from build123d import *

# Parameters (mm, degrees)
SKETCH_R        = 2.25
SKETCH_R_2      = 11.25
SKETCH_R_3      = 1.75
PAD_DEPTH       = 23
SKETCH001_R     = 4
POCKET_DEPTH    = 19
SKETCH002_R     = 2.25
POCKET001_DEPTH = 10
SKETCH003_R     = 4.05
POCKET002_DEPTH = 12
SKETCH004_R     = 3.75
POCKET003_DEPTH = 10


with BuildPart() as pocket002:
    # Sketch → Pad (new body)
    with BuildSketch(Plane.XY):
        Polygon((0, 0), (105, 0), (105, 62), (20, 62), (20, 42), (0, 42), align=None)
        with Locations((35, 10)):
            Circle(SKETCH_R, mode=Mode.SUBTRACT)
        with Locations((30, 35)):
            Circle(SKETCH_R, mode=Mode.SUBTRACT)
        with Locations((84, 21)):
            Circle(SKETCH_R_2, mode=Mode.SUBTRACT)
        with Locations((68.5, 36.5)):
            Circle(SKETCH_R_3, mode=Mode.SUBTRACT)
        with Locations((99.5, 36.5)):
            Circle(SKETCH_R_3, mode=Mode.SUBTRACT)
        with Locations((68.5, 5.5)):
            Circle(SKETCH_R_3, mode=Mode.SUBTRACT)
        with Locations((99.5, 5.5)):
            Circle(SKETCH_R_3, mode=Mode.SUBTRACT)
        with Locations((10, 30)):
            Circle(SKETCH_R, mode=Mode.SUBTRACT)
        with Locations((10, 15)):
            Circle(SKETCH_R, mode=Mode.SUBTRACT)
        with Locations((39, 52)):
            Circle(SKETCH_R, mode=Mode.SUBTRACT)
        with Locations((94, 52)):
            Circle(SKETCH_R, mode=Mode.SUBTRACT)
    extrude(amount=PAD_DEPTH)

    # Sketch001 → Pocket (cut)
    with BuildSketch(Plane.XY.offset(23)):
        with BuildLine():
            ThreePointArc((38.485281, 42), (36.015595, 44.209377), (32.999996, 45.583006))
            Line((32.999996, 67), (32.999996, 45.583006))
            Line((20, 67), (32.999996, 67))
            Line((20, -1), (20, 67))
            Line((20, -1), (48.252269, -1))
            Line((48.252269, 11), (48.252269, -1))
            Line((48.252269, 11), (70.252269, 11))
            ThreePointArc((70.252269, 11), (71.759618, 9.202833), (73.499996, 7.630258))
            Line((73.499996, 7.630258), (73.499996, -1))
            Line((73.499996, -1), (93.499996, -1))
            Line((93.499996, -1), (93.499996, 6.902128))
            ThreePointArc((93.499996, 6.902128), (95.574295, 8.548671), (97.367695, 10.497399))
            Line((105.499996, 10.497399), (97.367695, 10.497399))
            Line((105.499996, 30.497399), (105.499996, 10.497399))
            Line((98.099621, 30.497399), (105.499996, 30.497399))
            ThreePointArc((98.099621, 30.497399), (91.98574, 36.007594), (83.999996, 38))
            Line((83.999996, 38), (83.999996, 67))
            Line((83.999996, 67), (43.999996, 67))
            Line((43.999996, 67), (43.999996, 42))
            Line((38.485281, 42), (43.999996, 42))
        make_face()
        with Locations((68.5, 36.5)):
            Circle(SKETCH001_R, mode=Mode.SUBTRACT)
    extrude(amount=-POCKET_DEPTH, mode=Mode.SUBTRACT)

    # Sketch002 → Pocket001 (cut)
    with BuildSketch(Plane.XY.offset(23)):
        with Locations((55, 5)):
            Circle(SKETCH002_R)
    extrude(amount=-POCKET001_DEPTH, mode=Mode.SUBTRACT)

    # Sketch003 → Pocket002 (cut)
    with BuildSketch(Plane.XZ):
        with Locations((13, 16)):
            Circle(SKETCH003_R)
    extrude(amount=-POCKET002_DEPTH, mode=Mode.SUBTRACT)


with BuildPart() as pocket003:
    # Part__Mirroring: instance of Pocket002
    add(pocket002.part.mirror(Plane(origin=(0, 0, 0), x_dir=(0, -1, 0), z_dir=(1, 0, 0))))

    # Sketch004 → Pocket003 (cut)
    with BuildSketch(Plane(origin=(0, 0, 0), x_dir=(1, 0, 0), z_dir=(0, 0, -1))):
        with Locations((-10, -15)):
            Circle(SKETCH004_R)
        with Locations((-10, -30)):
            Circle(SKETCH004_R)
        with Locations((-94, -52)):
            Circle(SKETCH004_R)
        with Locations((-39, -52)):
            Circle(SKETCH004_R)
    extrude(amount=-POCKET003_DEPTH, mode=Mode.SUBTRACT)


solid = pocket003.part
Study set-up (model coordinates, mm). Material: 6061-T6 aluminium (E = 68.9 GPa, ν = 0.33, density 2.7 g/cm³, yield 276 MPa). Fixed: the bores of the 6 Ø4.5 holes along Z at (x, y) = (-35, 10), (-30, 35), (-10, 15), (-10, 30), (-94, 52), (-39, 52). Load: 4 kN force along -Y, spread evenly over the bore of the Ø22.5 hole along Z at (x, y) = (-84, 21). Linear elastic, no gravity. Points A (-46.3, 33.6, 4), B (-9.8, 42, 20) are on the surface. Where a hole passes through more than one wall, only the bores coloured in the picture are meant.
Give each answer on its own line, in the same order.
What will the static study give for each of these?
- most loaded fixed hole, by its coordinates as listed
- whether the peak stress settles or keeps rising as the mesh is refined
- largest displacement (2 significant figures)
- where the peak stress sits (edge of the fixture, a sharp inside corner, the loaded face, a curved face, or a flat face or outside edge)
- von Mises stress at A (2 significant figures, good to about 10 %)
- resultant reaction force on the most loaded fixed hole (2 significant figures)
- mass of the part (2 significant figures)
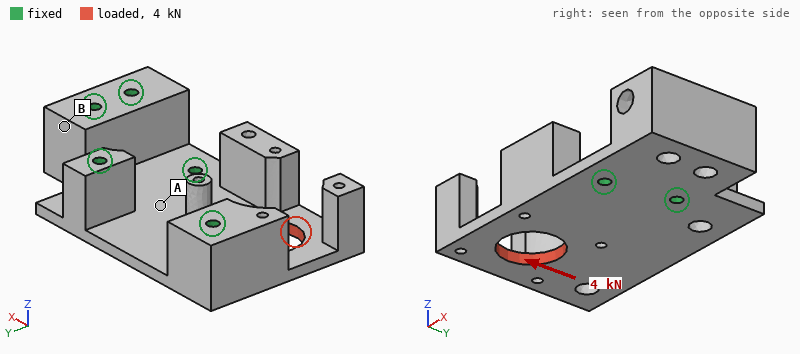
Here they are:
(-94, 52)
keeps rising
51 µm
edge of the fixture
13 MPa
2.6 kN
160 g
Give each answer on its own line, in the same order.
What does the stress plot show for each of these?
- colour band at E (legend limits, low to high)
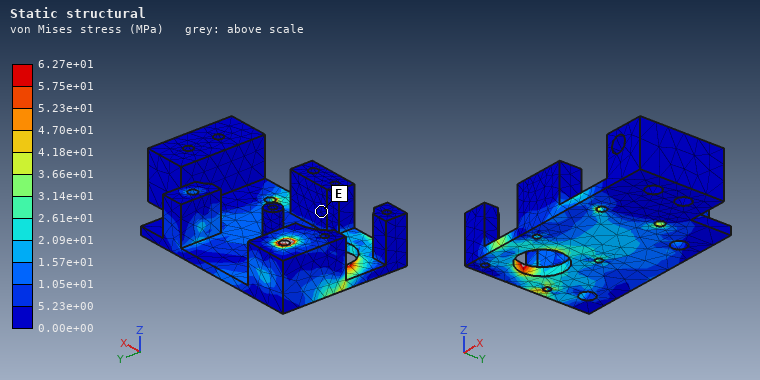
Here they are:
0.00e+00 to 5.23e+00 MPa
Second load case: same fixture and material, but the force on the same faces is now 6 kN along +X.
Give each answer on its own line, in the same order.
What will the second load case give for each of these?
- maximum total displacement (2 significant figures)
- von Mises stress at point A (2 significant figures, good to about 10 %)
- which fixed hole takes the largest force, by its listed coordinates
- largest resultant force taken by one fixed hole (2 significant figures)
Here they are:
42 µm
22 MPa
(-35, 10)
2.4 kN
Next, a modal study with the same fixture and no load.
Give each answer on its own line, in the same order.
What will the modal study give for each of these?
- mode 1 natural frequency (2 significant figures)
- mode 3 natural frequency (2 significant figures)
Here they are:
1600 Hz
4300 Hz
